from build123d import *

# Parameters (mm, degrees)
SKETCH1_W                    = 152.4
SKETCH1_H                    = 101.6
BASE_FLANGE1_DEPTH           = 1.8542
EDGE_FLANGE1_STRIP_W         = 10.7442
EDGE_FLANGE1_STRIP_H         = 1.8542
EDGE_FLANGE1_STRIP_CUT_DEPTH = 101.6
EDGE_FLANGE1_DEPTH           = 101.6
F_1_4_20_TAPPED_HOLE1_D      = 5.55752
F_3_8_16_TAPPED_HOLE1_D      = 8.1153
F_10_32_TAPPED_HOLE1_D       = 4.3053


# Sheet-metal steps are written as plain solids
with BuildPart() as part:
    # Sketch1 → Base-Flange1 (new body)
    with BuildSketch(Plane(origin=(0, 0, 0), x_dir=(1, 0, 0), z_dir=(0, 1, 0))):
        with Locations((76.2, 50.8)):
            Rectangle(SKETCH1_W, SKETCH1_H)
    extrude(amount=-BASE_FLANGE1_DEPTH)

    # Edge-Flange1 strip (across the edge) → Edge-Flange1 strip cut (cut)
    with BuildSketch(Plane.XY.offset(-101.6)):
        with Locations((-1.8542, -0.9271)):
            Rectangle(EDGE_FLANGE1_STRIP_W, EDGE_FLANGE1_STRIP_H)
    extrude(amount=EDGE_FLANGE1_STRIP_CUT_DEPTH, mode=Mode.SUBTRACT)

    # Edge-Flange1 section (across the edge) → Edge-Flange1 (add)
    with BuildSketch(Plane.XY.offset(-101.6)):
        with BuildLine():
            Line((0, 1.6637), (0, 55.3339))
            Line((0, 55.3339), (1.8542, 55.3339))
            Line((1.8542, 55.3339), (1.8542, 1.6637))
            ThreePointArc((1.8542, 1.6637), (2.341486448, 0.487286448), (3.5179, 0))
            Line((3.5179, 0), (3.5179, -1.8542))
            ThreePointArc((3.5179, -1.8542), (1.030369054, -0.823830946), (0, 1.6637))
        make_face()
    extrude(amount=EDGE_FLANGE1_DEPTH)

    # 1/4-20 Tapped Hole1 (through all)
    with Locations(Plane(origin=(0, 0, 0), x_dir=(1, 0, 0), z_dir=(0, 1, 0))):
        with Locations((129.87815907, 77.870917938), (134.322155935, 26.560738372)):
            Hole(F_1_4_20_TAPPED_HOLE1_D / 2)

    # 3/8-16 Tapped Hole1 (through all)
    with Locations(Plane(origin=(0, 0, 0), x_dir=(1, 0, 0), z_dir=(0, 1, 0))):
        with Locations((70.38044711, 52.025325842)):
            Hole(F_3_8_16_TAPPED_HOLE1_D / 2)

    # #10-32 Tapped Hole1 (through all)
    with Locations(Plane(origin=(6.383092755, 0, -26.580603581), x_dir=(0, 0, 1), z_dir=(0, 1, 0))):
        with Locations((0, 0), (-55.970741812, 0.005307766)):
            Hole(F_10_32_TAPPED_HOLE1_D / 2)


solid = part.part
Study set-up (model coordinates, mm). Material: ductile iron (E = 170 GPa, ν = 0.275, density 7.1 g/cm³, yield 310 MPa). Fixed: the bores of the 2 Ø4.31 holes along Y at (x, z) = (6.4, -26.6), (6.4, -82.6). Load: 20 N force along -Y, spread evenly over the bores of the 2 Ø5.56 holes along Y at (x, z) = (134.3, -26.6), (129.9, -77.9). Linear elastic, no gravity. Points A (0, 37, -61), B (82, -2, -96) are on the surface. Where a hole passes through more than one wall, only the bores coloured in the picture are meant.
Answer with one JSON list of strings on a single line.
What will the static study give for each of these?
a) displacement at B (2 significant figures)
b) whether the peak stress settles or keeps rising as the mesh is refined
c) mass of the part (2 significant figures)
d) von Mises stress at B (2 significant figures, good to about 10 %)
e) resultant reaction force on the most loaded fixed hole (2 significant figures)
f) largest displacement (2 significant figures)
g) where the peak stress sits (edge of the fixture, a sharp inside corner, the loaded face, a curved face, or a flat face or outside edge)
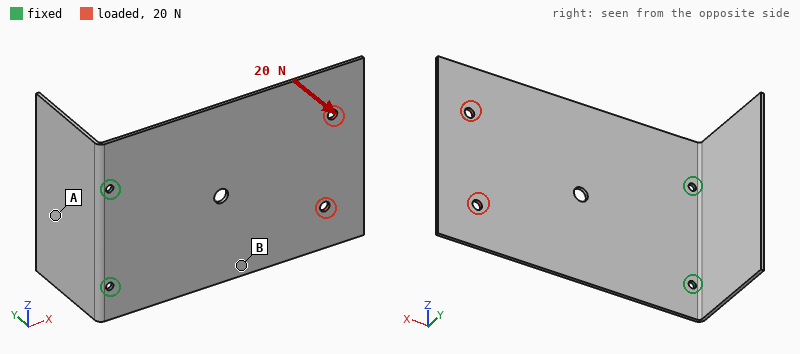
["0.64 mm", "keeps rising", "270 g", "18 MPa", "13 N", "1.8 mm", "edge of the fixture"]
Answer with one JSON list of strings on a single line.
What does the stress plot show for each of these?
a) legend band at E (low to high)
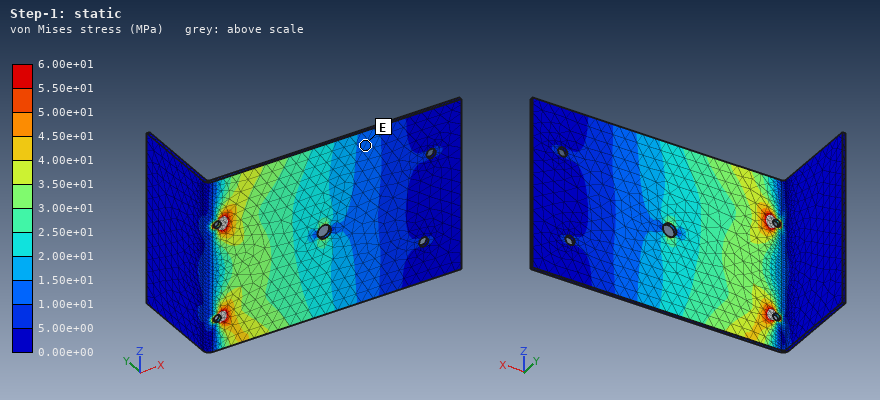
["1.00e+01 to 1.50e+01 MPa"]
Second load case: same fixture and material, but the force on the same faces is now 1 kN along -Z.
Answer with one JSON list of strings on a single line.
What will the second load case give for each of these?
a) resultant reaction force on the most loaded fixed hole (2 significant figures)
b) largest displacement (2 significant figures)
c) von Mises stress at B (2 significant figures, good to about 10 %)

["2.2 kN", "77 µm", "14 MPa"]
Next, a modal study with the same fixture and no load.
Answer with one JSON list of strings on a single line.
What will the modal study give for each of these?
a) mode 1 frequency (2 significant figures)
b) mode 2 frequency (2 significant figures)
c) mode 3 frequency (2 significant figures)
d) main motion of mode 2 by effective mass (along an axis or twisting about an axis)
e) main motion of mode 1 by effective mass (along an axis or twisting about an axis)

["68 Hz", "220 Hz", "380 Hz", "twisting about X", "along Y"]
